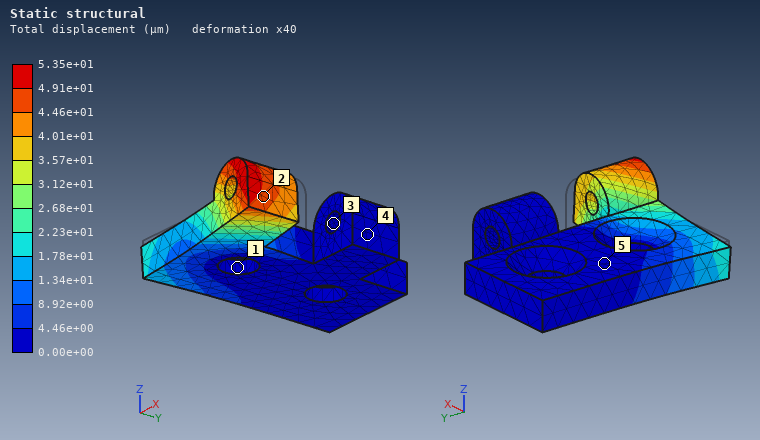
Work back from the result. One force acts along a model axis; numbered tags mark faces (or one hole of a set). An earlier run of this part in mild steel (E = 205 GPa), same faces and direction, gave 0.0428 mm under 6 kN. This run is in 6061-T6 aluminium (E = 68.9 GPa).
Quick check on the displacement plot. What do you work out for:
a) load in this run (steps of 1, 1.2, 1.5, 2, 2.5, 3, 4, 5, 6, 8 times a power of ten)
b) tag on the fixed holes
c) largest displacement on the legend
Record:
2.5 kN
1
5.35e+01 µm
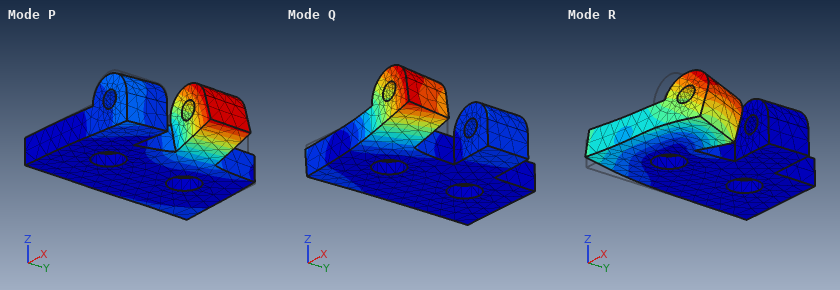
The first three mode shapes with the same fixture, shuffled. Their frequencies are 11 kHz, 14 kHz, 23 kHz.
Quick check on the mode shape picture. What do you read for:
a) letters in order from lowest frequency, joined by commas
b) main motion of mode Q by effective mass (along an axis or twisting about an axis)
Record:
Q, P, R
along Z
